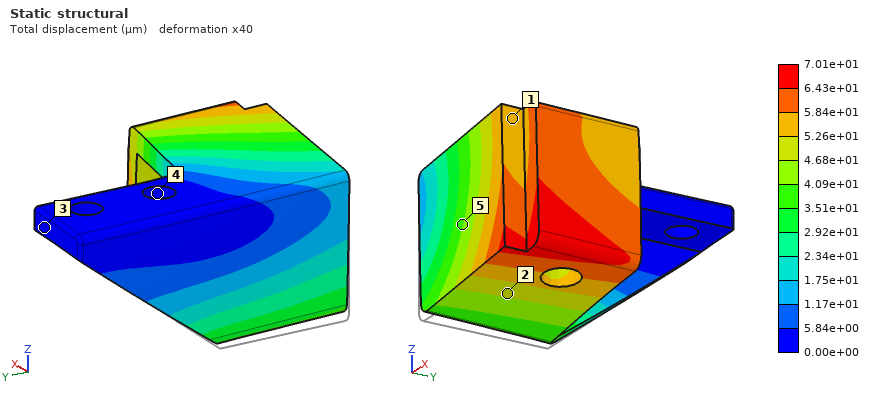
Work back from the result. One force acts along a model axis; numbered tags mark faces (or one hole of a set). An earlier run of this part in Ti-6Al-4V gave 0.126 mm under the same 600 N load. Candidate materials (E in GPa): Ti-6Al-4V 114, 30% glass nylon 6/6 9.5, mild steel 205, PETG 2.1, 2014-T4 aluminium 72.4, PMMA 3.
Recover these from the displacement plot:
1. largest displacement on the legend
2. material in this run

7.01e+01 µm
mild steel
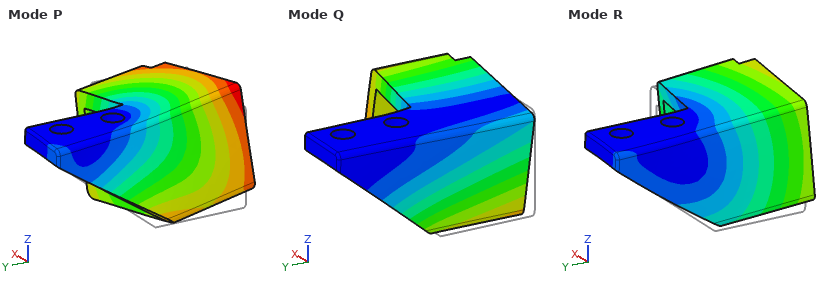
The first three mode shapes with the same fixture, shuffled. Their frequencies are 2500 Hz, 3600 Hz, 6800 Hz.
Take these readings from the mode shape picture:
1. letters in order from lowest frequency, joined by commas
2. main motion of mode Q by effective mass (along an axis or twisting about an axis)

Q, R, P
along X
